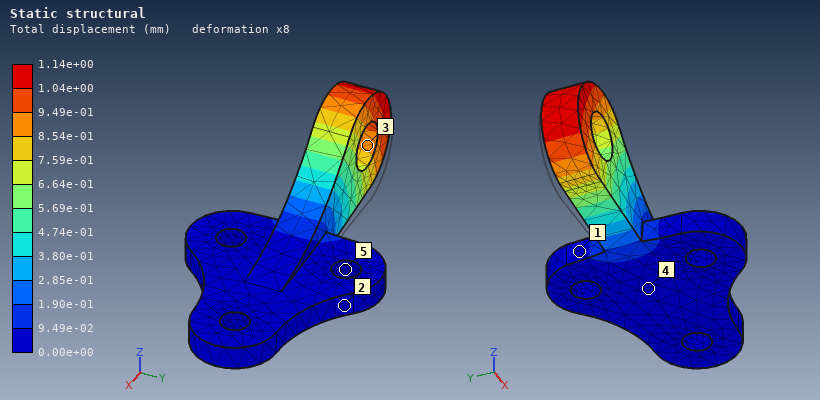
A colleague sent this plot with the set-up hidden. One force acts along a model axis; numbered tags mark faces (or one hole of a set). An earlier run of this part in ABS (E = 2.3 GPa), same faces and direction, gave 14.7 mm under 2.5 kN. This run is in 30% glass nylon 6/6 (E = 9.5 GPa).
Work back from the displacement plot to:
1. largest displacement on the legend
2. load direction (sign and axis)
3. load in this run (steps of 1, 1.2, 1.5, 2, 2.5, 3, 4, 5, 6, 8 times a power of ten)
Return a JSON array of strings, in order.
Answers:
["1.14e+00 mm", "+Z", "800 N"]
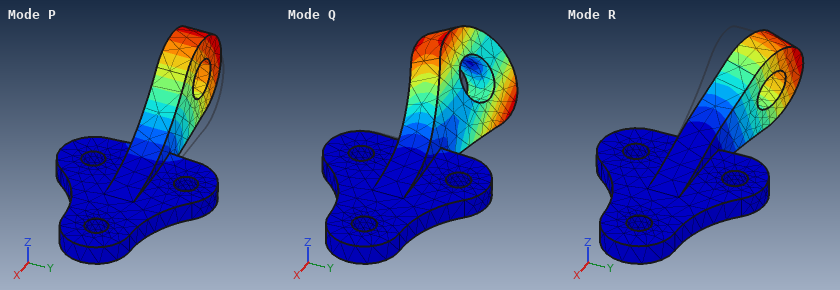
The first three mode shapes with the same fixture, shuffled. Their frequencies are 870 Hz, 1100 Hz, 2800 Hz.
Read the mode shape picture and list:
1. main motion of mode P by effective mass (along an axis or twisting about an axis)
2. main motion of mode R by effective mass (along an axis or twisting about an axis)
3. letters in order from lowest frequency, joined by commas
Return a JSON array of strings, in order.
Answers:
["along Z", "along Y", "P, R, Q"]
